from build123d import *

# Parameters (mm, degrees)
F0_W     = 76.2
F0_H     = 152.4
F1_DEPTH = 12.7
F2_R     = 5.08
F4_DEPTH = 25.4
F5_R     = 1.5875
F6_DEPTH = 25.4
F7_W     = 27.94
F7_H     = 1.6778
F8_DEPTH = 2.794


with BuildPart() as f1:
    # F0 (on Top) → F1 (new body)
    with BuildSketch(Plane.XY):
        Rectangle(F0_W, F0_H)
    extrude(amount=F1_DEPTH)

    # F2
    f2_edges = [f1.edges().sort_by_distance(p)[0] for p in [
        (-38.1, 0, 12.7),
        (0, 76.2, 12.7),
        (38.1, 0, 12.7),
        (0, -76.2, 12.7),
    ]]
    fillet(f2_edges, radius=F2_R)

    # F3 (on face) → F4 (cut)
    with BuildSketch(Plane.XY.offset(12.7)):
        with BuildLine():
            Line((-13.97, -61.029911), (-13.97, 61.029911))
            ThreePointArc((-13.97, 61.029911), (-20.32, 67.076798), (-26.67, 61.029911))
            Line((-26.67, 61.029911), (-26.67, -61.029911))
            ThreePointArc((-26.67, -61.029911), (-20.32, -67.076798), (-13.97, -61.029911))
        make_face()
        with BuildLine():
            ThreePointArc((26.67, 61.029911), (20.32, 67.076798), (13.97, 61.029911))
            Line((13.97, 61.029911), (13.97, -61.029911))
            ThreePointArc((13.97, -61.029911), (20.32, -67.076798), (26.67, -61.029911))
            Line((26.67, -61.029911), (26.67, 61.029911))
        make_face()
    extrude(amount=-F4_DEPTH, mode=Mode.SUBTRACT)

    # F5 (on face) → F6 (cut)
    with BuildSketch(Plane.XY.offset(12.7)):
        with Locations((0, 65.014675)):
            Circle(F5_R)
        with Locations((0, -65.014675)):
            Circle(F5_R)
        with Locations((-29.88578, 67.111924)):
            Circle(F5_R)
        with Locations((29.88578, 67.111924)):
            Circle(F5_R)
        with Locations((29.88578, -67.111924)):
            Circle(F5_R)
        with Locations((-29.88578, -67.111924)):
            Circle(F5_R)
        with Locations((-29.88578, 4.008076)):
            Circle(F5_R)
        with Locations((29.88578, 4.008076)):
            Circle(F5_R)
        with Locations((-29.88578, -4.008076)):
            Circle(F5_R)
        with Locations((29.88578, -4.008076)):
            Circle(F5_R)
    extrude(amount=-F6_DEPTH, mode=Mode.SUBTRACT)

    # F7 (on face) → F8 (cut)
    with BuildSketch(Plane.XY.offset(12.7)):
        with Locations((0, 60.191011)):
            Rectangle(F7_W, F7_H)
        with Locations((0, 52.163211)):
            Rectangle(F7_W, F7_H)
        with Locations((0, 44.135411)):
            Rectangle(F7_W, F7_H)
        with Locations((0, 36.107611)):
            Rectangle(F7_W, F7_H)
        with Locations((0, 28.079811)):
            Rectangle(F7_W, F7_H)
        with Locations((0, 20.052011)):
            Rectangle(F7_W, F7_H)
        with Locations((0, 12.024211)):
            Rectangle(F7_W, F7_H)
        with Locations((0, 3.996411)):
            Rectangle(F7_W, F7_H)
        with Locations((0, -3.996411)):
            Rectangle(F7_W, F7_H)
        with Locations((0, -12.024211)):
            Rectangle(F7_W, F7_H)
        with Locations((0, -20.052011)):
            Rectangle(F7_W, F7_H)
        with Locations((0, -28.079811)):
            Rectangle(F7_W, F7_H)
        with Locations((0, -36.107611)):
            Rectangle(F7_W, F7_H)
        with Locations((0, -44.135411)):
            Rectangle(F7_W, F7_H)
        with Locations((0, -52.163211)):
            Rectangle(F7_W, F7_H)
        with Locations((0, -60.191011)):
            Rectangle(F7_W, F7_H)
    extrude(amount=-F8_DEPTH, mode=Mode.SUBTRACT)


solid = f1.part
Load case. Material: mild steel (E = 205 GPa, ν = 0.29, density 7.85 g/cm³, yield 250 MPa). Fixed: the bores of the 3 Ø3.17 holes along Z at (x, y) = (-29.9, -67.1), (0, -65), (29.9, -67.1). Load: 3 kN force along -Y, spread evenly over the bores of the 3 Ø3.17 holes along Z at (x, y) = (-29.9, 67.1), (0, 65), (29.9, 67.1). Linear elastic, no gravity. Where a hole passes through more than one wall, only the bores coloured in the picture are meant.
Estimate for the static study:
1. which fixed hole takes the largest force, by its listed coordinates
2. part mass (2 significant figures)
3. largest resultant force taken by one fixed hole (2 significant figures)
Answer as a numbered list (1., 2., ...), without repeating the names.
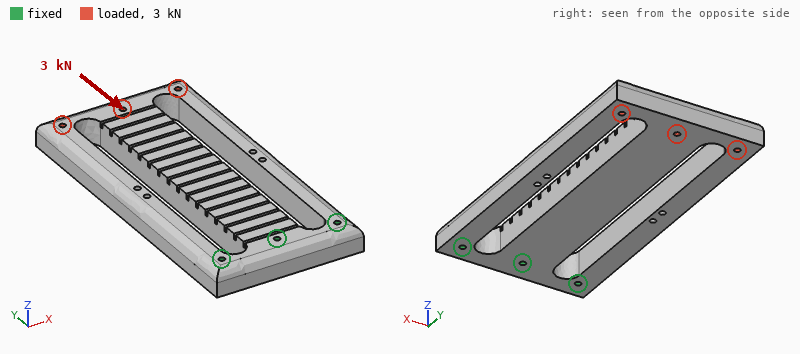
1. (0, -65)
2. 780 g
3. 1.2 kN
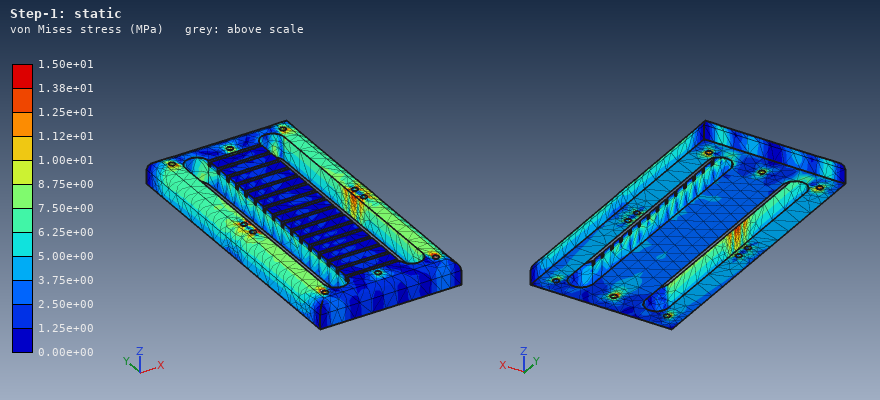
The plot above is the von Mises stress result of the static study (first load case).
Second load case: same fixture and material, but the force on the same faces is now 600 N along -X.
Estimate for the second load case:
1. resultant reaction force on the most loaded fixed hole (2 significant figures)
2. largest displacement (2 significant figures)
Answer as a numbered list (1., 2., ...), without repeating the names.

1. 1.2 kN
2. 52 µm
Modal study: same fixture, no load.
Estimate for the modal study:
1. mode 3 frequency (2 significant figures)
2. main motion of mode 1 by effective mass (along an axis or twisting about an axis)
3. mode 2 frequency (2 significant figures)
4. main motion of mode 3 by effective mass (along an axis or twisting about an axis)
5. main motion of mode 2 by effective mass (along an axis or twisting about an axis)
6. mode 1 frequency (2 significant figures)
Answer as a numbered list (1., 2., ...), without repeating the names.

1. 1400 Hz
2. along Z
3. 990 Hz
4. twisting about Y
5. along X
6. 420 Hz
